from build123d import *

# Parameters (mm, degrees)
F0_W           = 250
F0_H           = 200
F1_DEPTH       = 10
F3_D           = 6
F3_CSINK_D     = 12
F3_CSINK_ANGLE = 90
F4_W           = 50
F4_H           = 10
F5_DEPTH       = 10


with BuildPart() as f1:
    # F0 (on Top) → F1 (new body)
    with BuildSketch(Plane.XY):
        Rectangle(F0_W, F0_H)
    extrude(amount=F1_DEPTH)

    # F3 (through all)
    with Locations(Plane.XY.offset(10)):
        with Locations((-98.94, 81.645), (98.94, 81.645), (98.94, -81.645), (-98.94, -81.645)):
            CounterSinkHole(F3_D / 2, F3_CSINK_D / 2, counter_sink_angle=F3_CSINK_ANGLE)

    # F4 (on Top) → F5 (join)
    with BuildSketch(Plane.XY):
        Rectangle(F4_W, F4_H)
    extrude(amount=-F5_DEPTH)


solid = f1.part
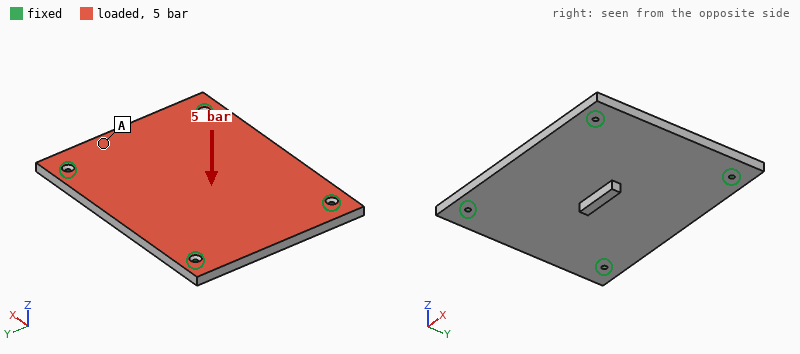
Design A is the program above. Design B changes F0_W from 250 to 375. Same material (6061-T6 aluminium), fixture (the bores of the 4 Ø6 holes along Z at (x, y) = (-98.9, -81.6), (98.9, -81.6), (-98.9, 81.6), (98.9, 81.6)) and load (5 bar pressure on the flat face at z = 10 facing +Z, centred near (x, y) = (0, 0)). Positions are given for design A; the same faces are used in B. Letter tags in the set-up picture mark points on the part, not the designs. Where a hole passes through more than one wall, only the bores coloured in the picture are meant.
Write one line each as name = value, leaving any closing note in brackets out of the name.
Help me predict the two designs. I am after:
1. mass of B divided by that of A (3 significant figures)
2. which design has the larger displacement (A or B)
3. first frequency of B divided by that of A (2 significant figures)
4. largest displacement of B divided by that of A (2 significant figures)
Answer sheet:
mass of B divided by that of A = 1.50
which design has the larger displacement = B
first frequency of B divided by that of A = 0.73
largest displacement of B divided by that of A = 1.6
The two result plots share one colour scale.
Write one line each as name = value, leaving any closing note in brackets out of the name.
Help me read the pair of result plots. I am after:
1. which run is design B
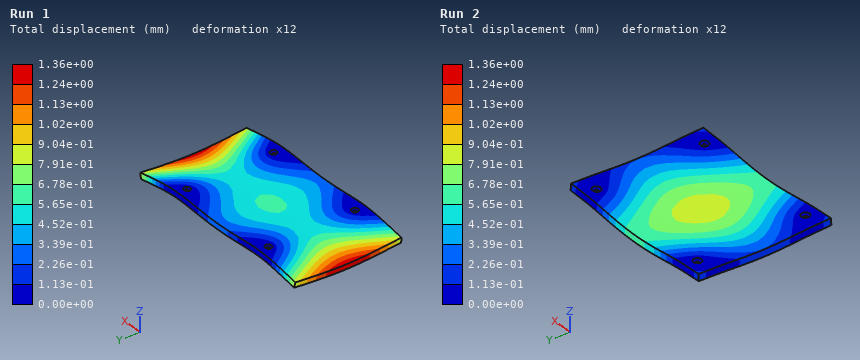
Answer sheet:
which run is design B = Run 1
